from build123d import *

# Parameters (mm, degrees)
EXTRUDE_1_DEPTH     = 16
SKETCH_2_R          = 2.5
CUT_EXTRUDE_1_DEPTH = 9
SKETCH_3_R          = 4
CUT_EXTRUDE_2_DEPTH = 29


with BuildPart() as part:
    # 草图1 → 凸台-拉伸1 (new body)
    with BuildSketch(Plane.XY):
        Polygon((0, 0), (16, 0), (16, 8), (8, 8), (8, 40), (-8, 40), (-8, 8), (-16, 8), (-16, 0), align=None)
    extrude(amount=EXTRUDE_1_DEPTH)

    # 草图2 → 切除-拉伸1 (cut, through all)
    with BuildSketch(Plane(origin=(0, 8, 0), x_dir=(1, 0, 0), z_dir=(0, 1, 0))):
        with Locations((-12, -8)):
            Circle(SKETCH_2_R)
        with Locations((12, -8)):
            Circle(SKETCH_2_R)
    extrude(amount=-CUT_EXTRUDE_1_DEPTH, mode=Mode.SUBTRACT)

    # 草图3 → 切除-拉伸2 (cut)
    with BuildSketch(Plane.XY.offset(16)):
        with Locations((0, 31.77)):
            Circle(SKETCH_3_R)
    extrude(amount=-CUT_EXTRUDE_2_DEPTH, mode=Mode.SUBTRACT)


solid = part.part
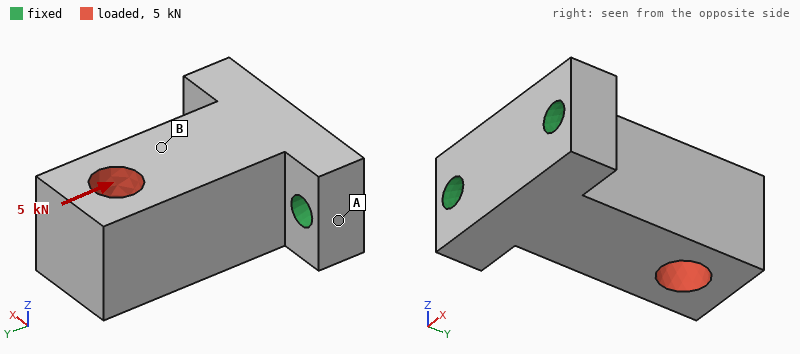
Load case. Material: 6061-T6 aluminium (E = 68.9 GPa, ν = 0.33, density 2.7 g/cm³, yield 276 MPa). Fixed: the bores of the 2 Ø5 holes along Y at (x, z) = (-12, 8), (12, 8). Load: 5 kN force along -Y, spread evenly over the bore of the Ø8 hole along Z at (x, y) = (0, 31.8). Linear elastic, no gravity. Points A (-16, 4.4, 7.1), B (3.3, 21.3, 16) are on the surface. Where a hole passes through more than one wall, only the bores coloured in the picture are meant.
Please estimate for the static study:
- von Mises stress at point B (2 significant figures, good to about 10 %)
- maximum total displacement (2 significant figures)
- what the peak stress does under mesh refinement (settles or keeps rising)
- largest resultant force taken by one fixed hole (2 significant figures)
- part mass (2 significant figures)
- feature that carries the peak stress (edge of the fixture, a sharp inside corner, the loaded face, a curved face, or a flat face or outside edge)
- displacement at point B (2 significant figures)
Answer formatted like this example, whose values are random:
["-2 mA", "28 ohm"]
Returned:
["18 MPa", "18 µm", "keeps rising", "2.6 kN", "30 g", "edge of the fixture", "10 µm"]
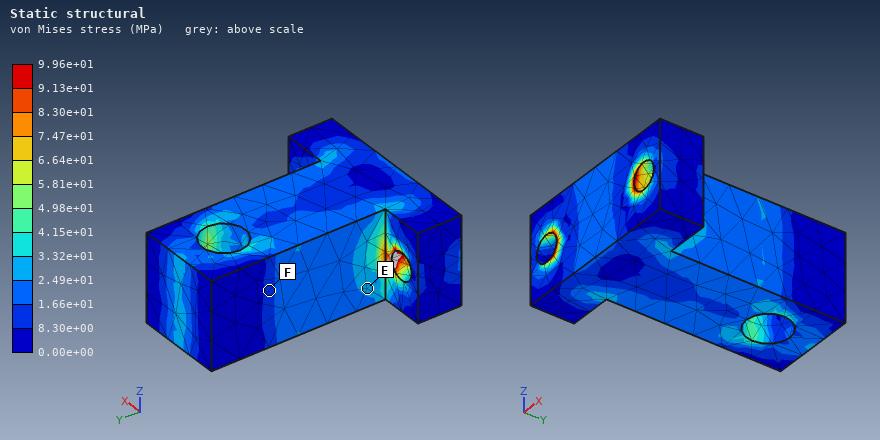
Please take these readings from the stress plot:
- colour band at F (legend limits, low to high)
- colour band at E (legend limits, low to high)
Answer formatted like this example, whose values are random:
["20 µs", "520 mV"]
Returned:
["8.30e+00 to 1.66e+01 MPa", "2.49e+01 to 3.32e+01 MPa"]
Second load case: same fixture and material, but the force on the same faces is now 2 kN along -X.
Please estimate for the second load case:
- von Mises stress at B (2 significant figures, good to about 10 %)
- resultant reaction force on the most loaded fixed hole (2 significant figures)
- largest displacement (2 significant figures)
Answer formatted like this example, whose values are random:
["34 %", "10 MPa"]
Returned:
["22 MPa", "2.9 kN", "79 µm"]
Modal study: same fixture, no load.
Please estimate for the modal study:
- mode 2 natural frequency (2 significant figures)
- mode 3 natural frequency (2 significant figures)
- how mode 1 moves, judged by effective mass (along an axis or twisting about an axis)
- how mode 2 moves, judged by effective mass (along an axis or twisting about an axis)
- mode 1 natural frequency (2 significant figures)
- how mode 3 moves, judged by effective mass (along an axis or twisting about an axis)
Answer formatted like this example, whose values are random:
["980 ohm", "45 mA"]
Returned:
["9000 Hz", "20 kHz", "along Z", "along X", "5900 Hz", "twisting about Y"]
